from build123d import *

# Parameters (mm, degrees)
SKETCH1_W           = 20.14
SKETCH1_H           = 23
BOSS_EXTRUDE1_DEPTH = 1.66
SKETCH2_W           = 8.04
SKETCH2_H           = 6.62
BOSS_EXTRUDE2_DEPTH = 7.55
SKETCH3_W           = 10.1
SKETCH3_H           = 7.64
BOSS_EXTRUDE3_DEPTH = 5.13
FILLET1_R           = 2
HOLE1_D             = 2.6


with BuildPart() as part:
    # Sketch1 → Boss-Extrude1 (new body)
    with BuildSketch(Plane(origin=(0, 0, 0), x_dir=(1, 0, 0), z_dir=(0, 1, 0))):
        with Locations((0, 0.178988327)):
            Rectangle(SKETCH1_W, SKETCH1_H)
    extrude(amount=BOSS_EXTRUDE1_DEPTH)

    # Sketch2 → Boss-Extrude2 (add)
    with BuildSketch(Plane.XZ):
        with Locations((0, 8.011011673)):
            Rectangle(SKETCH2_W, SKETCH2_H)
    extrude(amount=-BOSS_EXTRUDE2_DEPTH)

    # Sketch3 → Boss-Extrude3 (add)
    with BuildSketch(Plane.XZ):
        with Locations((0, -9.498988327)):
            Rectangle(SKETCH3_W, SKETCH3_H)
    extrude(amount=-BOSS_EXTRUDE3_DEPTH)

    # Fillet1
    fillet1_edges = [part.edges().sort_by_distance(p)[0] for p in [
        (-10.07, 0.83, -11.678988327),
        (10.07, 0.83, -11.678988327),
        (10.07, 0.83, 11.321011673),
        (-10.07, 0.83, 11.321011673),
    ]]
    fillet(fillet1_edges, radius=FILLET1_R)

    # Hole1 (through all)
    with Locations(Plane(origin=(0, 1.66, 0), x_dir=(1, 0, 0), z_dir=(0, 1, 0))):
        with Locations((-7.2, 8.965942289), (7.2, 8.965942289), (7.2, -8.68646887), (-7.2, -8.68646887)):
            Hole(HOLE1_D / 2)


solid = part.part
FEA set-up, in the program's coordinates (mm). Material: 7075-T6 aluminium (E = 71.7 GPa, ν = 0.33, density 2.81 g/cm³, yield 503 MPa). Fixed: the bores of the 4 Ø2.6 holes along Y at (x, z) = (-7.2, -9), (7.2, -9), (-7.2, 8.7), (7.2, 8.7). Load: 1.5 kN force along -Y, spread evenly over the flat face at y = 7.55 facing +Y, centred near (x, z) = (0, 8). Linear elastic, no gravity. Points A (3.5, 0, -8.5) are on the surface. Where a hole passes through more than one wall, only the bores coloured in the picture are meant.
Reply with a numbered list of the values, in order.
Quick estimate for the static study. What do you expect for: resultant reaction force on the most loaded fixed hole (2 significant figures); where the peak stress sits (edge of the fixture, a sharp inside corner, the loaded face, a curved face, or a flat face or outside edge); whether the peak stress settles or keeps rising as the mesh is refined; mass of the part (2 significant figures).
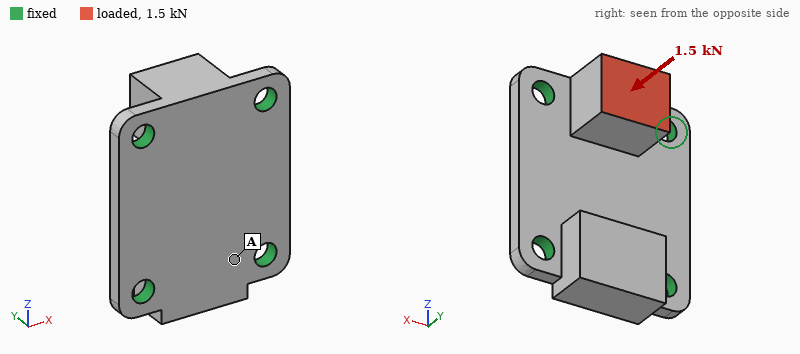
1. 780 N
2. edge of the fixture
3. keeps rising
4. 3.8 g
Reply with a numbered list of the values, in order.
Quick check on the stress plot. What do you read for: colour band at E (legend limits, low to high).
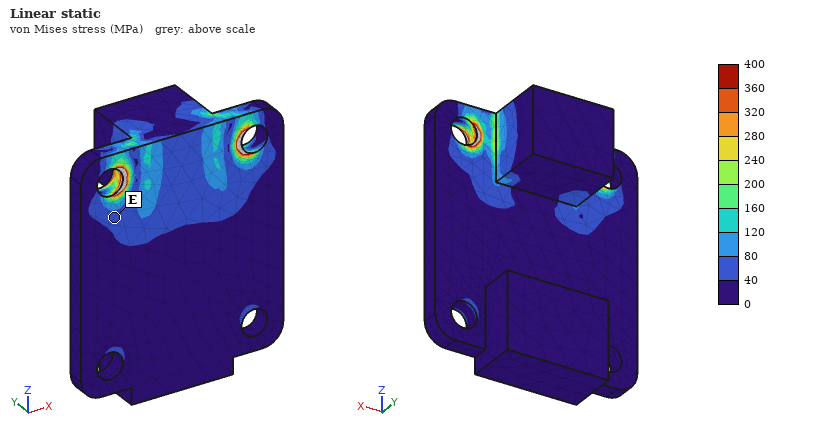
1. 40 to 80 MPa
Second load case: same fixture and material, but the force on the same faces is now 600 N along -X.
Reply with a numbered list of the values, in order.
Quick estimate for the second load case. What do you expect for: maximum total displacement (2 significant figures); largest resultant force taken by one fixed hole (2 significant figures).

1. 21 µm
2. 460 N
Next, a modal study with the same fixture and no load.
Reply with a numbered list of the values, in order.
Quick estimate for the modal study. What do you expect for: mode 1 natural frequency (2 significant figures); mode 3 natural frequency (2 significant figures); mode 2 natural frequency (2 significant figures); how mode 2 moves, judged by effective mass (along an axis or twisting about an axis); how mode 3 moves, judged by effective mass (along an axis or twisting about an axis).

1. 20 kHz
2. 37 kHz
3. 30 kHz
4. along Z
5. twisting about Z
